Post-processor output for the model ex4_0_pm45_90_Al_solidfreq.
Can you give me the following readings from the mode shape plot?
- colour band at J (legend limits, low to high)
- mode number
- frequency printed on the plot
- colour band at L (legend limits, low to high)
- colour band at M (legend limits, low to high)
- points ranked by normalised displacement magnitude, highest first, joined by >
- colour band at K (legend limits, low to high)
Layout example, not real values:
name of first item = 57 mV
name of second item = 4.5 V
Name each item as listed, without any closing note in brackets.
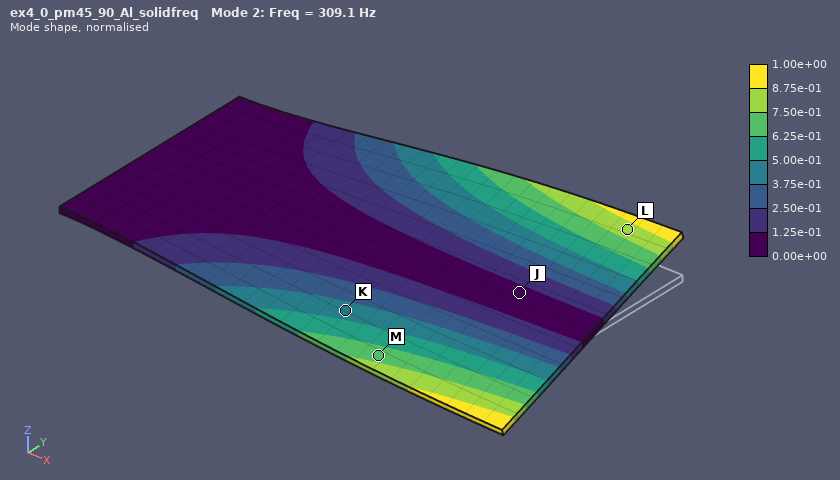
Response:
colour band at J = 0.00e+00 to 1.25e-01
mode number = 2
frequency printed on the plot = 309.1 Hz
colour band at L = 7.50e-01 to 8.75e-01
colour band at M = 6.25e-01 to 7.50e-01
points ranked by normalised displacement magnitude, highest first, joined by > = L > M > K > J
colour band at K = 3.75e-01 to 5.00e-01
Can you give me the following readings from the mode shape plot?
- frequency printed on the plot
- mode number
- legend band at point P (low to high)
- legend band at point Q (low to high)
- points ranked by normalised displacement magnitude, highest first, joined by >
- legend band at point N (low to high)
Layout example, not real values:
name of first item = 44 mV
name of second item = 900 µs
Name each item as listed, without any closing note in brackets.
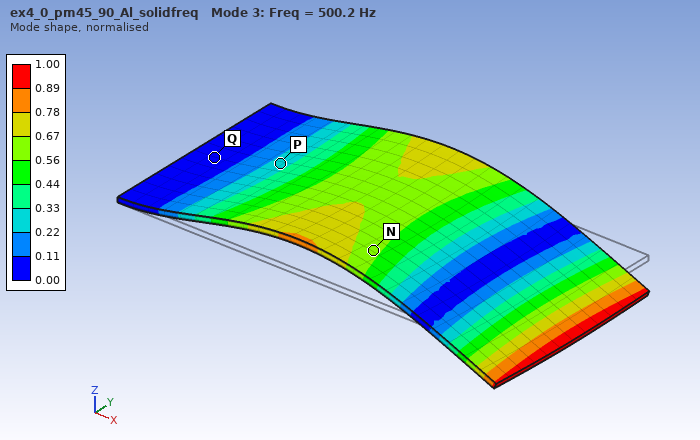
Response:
frequency printed on the plot = 500.2 Hz
mode number = 3
legend band at point P = 0.22 to 0.33
legend band at point Q = 0.00 to 0.11
points ranked by normalised displacement magnitude, highest first, joined by > = N > P > Q
legend band at point N = 0.56 to 0.67
